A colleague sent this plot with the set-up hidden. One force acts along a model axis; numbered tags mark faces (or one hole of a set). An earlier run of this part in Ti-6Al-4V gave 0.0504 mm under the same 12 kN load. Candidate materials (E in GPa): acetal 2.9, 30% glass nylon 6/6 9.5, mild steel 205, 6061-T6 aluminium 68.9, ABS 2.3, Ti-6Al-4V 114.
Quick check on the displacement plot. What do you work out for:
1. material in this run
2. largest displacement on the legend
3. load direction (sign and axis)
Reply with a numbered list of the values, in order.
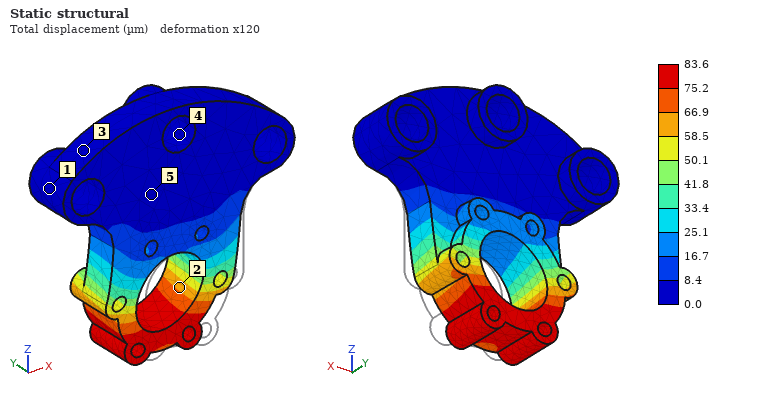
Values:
1. 6061-T6 aluminium
2. 83.6 µm
3. -X
